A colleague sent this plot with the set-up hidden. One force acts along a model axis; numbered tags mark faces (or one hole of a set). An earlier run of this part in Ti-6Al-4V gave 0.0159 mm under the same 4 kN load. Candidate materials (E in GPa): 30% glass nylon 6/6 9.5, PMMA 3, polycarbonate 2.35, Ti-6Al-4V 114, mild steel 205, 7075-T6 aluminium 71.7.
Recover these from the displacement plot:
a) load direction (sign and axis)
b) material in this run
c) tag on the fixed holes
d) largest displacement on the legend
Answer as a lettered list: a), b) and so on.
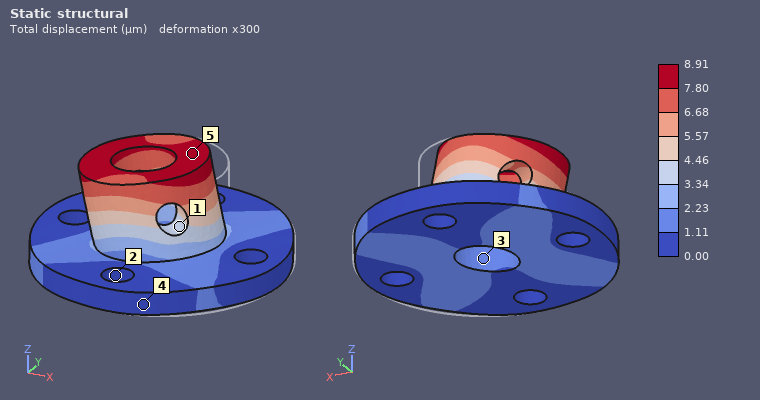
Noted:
a) -X
b) mild steel
c) 2
d) 8.91 µm
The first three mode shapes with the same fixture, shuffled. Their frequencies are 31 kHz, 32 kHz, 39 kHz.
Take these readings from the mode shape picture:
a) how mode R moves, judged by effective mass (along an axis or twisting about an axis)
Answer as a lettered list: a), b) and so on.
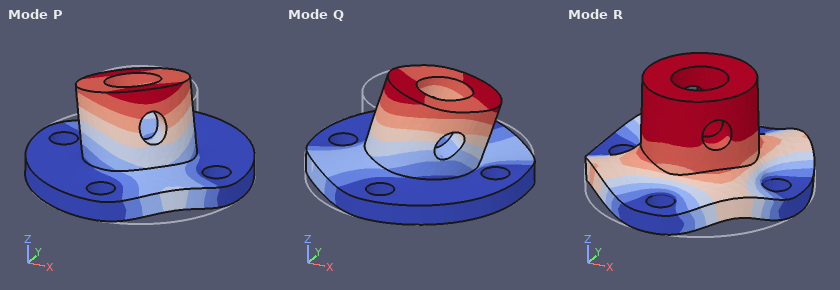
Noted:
a) along Z
